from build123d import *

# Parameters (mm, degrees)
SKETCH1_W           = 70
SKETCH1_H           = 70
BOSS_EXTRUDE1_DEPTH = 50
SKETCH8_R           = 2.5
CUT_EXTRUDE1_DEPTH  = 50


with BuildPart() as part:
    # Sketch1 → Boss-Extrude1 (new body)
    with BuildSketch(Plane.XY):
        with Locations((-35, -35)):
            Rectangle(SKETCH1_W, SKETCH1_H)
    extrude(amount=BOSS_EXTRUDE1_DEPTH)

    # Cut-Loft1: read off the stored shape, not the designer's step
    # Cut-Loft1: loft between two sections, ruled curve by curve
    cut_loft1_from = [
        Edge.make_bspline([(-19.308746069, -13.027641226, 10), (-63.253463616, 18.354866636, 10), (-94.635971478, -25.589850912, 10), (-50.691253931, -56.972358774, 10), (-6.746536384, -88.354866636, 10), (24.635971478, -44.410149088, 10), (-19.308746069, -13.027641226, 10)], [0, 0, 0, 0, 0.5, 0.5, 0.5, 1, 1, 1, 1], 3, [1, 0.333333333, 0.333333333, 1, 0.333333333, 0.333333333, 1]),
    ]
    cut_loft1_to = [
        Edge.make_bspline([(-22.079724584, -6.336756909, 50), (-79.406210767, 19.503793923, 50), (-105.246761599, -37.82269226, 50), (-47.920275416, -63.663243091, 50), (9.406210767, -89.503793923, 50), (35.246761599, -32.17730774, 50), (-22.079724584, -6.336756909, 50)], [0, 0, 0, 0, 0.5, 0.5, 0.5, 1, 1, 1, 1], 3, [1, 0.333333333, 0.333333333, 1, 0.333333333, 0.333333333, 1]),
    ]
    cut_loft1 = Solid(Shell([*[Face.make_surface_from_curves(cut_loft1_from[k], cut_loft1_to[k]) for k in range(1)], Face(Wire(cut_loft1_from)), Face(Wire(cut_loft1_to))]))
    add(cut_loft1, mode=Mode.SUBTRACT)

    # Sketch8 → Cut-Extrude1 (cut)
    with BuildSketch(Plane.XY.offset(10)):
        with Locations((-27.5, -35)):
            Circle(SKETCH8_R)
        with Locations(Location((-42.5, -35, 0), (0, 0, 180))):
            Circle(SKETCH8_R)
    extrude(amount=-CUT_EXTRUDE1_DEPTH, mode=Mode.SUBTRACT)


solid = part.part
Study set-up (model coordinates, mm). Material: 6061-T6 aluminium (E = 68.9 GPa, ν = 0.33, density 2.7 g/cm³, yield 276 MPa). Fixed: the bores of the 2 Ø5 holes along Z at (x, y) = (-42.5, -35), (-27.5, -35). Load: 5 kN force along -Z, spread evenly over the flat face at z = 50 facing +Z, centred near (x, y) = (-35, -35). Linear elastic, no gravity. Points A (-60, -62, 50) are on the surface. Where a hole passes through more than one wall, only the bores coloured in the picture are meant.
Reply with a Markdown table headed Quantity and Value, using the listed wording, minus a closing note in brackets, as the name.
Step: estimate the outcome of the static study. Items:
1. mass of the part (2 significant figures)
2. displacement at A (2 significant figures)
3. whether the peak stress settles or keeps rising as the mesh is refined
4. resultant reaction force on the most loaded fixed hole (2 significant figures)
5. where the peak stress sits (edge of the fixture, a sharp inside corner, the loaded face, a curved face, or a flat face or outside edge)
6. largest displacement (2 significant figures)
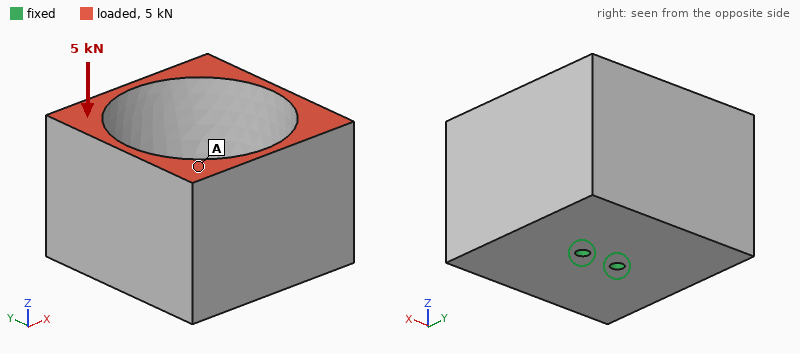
| Quantity | Value |
|---|---|
| mass of the part | 370 g |
| displacement at A | 18 µm |
| whether the peak stress settles or keeps rising as the mesh is refined | keeps rising |
| resultant reaction force on the most loaded fixed hole | 2.5 kN |
| where the peak stress sits | edge of the fixture |
| largest displacement | 18 µm |
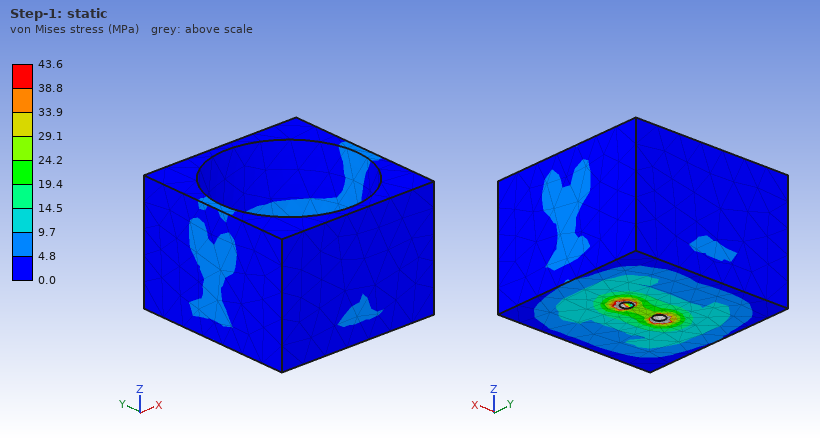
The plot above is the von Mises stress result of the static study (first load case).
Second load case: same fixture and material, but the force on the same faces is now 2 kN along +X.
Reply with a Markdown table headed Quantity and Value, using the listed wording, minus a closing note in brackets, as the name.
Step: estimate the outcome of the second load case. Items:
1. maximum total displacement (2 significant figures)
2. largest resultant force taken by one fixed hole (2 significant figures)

| Quantity | Value |
|---|---|
| maximum total displacement | 74 µm |
| largest resultant force taken by one fixed hole | 3.3 kN |
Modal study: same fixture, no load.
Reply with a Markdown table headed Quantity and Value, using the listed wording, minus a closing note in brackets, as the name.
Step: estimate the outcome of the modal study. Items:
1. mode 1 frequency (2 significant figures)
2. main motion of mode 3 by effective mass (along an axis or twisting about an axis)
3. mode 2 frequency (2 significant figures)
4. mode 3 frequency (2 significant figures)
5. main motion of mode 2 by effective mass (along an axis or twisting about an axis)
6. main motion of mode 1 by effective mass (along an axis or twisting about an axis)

| Quantity | Value |
|---|---|
| mode 1 frequency | 1700 Hz |
| main motion of mode 3 by effective mass | twisting about Z |
| mode 2 frequency | 2300 Hz |
| mode 3 frequency | 3200 Hz |
| main motion of mode 2 by effective mass | along X |
| main motion of mode 1 by effective mass | along Y |
